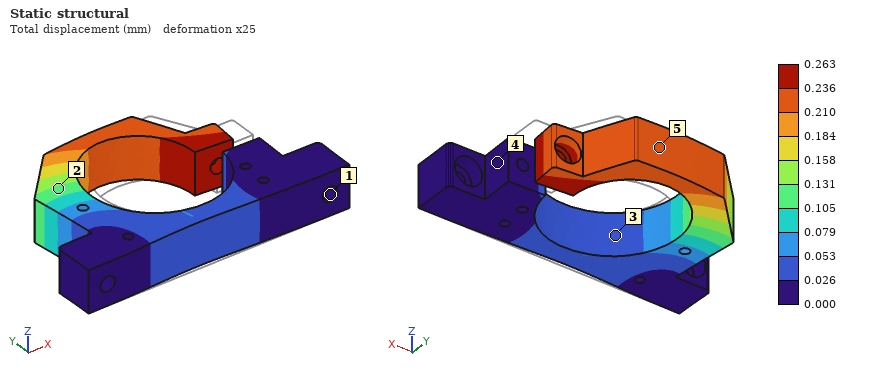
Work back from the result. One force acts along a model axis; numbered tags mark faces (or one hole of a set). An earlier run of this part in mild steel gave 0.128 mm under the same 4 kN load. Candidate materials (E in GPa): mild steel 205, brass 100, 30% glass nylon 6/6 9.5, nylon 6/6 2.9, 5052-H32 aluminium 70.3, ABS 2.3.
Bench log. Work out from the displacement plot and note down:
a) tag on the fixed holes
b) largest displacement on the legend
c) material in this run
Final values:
1
0.263 mm
brass
